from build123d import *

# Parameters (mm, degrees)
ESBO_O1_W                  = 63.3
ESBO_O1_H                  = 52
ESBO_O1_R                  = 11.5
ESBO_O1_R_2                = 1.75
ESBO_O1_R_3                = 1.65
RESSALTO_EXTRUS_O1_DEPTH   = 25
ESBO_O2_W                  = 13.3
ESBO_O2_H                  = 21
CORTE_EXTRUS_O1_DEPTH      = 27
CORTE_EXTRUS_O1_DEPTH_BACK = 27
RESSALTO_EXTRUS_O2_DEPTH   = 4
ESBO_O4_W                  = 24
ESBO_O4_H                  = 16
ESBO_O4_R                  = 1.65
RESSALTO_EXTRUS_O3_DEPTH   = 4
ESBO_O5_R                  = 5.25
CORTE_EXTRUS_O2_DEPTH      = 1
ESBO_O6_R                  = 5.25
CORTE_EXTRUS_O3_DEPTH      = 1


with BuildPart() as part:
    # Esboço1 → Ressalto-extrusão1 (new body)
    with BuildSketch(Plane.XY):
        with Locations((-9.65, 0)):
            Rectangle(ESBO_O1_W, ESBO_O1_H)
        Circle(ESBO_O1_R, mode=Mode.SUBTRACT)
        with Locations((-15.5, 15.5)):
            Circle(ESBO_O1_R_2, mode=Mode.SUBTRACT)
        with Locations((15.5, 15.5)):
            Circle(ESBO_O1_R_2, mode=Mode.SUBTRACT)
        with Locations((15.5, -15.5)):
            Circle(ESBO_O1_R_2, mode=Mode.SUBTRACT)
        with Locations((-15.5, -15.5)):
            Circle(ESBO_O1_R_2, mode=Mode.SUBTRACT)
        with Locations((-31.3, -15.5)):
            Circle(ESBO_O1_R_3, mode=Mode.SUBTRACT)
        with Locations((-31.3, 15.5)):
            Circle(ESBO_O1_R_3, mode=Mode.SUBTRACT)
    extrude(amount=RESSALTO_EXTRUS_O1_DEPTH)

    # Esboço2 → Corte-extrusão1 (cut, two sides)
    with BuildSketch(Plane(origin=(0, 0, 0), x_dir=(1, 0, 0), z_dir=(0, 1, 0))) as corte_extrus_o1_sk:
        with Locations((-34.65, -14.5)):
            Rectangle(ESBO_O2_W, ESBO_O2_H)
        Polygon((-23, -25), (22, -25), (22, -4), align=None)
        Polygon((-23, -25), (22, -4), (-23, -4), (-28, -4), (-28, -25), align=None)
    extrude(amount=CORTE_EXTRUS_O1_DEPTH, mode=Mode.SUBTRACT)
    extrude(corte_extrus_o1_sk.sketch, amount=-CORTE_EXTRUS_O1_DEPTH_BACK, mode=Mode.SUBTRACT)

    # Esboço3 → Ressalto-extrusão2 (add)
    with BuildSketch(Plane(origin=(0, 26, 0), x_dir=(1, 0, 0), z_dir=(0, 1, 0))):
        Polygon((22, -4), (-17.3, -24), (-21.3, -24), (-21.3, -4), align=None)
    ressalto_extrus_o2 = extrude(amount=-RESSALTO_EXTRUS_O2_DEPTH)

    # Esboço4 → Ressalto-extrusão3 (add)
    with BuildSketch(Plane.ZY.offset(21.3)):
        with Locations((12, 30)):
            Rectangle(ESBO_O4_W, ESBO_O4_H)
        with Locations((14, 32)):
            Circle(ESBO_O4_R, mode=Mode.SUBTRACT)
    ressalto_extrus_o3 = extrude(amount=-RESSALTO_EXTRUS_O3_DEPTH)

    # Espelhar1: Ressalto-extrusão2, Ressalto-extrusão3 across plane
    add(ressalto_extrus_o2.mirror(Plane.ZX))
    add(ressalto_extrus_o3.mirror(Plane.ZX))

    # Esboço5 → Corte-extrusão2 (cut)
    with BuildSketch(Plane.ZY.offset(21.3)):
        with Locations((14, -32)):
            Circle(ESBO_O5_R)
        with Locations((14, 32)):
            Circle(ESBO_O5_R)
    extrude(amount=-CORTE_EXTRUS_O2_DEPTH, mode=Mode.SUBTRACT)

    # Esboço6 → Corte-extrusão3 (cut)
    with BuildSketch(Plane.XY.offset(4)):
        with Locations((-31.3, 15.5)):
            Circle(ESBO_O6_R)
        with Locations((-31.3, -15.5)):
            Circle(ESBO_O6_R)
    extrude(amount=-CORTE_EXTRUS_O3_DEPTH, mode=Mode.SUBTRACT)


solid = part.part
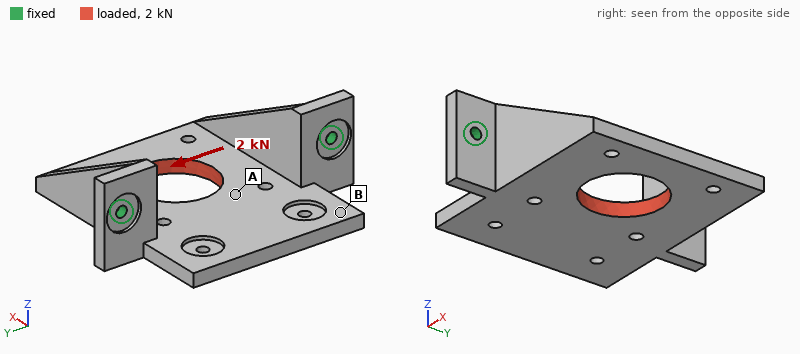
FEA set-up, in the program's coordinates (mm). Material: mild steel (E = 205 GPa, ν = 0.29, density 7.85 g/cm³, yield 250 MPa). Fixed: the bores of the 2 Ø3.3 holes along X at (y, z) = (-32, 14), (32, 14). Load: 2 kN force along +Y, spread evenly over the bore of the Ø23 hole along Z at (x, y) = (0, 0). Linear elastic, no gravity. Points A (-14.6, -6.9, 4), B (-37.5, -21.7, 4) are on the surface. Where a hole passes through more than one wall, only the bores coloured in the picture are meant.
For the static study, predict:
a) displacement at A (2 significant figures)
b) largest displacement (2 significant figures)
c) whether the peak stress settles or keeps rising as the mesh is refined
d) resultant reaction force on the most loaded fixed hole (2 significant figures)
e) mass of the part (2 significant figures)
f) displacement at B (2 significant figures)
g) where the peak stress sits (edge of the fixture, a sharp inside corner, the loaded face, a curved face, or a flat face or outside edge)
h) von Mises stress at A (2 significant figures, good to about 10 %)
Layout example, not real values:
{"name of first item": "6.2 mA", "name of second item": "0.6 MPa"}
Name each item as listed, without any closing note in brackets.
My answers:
{"displacement at A": "16 µm", "largest displacement": "55 µm", "whether the peak stress settles or keeps rising as the mesh is refined": "keeps rising", "resultant reaction force on the most loaded fixed hole": "1.2 kN", "mass of the part": "130 g", "displacement at B": "9.5 µm", "where the peak stress sits": "edge of the fixture", "von Mises stress at A": "43 MPa"}
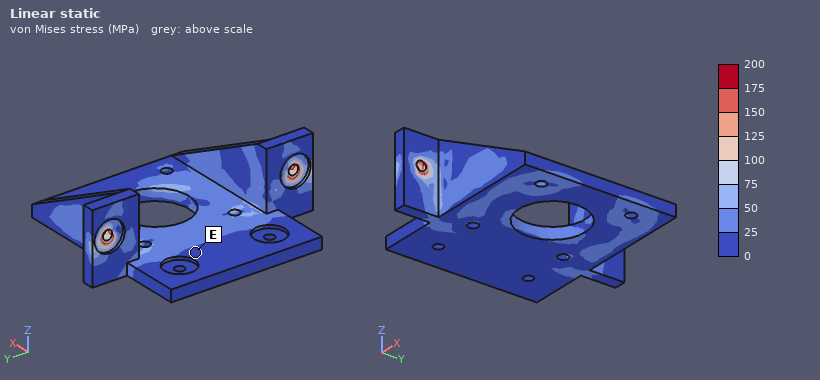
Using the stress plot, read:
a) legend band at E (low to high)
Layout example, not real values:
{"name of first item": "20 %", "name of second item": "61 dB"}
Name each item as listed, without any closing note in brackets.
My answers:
{"legend band at E": "0 to 25 MPa"}
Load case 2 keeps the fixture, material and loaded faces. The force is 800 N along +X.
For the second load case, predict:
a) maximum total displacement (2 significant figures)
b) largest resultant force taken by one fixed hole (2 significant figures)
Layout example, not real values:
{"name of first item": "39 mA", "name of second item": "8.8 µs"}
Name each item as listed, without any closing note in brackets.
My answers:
{"maximum total displacement": "70 µm", "largest resultant force taken by one fixed hole": "400 N"}
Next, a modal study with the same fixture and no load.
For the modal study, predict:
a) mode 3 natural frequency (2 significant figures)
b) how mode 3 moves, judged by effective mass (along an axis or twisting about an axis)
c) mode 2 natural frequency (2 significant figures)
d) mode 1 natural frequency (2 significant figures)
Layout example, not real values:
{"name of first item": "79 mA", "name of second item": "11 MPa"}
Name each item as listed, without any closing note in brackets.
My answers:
{"mode 3 natural frequency": "4000 Hz", "how mode 3 moves, judged by effective mass": "along Z", "mode 2 natural frequency": "3100 Hz", "mode 1 natural frequency": "1500 Hz"}
